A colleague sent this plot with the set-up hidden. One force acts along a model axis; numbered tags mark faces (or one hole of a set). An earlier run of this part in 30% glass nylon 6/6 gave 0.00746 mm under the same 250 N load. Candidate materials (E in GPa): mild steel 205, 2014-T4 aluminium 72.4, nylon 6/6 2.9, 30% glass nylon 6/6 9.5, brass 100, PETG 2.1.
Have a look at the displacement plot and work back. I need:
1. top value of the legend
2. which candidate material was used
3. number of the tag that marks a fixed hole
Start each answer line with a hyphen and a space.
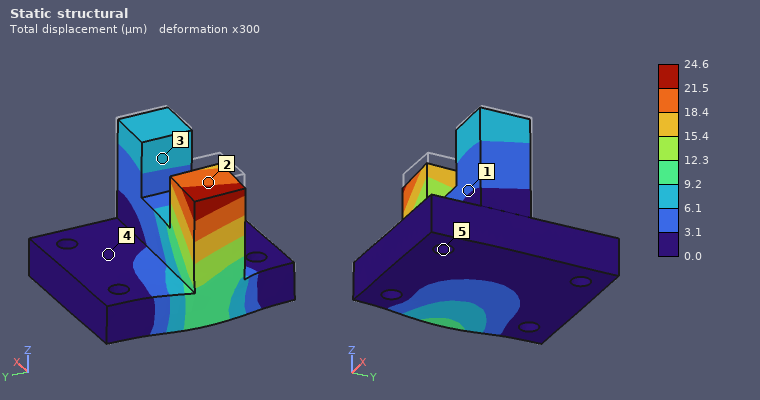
- 24.6 µm
- nylon 6/6
- 5
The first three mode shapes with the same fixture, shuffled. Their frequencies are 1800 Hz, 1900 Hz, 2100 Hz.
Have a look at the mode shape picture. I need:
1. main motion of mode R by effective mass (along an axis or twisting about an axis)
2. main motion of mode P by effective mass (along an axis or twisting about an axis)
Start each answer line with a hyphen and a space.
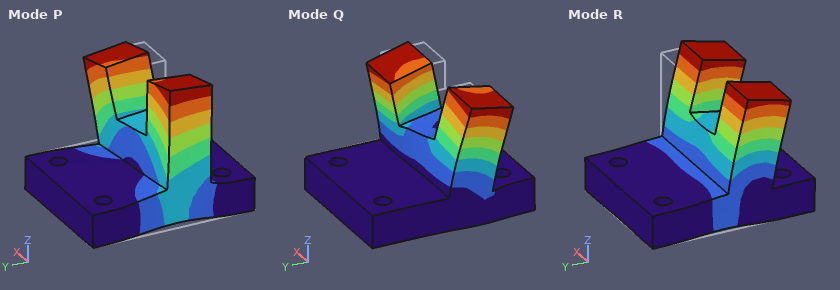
- along Y
- along X
